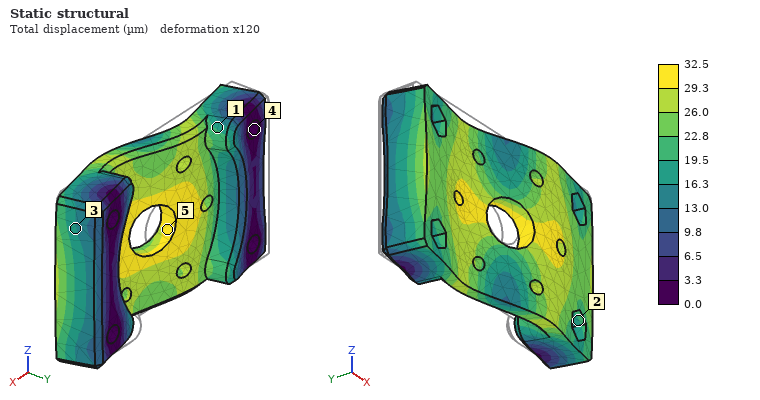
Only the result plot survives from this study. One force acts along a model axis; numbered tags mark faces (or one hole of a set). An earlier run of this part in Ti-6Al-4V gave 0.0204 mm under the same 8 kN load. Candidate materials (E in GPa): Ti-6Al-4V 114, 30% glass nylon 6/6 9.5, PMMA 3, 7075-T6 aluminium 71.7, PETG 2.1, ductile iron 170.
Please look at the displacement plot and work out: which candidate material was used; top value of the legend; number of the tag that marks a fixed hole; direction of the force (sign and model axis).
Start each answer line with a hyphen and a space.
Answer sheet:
- 7075-T6 aluminium
- 32.5 µm
- 4
- +X
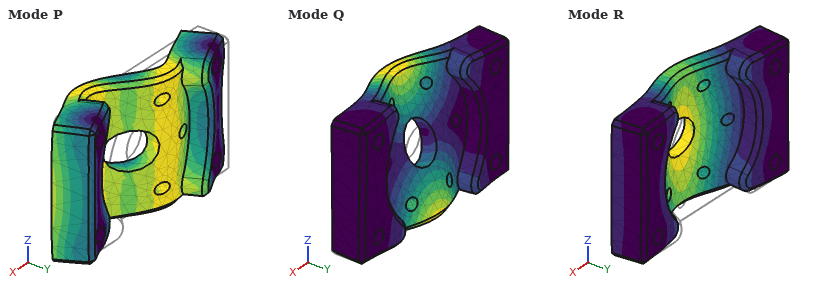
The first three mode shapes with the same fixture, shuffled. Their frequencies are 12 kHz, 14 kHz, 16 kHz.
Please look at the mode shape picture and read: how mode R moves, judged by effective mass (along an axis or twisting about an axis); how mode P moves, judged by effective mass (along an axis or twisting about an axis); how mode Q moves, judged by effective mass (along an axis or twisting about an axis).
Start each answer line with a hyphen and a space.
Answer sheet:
- along Y
- along X
- twisting about X
